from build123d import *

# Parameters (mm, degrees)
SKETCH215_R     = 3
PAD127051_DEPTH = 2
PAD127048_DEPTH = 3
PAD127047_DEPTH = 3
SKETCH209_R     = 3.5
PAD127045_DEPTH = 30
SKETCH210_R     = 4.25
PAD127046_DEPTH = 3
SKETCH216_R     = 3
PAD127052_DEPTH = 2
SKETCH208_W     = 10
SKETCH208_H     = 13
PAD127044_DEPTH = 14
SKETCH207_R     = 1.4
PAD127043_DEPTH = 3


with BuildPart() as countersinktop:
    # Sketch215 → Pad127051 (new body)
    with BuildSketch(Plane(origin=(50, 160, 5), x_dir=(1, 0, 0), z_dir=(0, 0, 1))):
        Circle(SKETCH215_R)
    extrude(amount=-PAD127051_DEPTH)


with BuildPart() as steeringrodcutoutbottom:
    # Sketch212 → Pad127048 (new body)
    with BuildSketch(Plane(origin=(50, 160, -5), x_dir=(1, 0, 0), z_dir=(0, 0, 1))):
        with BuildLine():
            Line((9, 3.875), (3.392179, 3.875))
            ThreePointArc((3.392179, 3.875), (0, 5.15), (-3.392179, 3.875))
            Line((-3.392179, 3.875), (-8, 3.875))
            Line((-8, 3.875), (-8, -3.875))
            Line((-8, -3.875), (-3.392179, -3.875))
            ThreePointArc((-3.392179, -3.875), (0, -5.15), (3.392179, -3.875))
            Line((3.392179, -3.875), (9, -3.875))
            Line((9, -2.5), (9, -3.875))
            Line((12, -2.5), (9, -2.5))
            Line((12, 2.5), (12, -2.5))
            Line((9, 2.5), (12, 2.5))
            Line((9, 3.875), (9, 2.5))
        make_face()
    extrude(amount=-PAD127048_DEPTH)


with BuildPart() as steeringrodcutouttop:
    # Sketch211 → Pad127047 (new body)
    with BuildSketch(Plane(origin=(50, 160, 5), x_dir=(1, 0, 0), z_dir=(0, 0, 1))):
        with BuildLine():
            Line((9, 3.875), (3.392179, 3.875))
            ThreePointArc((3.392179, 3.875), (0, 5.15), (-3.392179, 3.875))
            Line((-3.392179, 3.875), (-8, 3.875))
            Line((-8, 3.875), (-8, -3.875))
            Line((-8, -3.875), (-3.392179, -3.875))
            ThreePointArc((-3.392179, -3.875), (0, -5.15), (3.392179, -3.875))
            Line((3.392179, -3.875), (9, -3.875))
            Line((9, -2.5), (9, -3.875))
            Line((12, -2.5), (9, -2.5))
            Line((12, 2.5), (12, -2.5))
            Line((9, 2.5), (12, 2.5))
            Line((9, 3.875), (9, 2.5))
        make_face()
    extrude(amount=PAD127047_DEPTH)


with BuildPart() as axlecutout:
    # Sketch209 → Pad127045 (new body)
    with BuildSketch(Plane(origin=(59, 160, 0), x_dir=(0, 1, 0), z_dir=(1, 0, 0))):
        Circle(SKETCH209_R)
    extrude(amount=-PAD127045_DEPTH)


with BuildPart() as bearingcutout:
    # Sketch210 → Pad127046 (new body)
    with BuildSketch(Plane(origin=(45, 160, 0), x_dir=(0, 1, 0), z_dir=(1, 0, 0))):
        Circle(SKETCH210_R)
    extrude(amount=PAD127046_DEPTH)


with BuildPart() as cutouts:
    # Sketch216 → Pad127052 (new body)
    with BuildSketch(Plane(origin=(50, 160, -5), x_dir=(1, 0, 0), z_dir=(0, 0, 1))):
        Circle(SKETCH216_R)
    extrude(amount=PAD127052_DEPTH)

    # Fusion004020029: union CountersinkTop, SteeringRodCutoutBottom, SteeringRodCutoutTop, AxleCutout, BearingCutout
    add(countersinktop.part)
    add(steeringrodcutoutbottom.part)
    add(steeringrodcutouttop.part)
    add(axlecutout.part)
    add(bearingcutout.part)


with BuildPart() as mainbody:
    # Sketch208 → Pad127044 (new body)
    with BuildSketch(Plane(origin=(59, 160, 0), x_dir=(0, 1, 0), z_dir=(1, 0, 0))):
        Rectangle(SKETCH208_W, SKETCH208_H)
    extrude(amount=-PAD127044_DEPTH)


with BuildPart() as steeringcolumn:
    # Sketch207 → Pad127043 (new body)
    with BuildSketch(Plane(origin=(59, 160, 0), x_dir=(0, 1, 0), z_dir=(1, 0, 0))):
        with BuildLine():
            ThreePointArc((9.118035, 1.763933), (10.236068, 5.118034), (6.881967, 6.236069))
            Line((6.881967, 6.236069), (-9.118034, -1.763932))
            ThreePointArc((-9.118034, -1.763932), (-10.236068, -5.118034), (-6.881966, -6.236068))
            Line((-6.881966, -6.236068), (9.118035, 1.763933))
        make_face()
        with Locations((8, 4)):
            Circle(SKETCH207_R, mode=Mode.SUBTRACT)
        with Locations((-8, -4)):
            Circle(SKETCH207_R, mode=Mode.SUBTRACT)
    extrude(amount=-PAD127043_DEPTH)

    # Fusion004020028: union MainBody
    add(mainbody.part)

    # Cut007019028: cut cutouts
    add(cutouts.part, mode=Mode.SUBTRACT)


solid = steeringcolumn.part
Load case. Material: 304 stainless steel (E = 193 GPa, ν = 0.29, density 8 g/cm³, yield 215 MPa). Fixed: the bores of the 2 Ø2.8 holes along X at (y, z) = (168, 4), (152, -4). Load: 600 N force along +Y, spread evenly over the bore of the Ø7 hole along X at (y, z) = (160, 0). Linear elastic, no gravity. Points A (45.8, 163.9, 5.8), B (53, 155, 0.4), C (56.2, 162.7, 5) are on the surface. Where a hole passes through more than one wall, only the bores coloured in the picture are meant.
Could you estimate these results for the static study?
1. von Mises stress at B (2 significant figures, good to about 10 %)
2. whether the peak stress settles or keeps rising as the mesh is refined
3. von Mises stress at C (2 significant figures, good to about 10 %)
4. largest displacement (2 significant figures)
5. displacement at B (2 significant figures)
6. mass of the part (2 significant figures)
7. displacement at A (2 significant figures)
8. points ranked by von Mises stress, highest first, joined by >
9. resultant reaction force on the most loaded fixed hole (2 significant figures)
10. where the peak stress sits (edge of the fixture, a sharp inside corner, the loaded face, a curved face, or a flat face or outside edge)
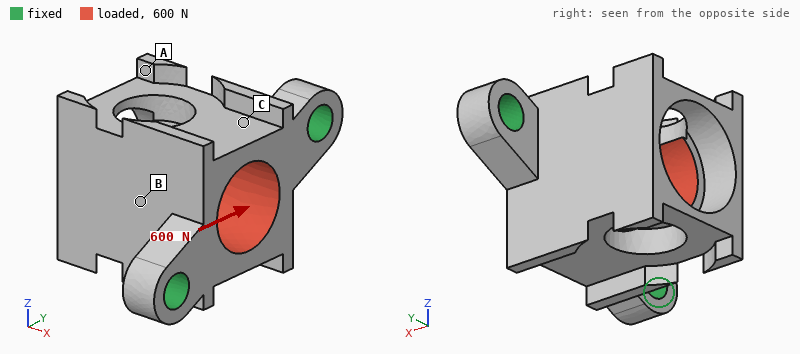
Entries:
19 MPa
keeps rising
40 MPa
12 µm
5.1 µm
7.2 g
10 µm
C > B > A
330 N
edge of the fixture
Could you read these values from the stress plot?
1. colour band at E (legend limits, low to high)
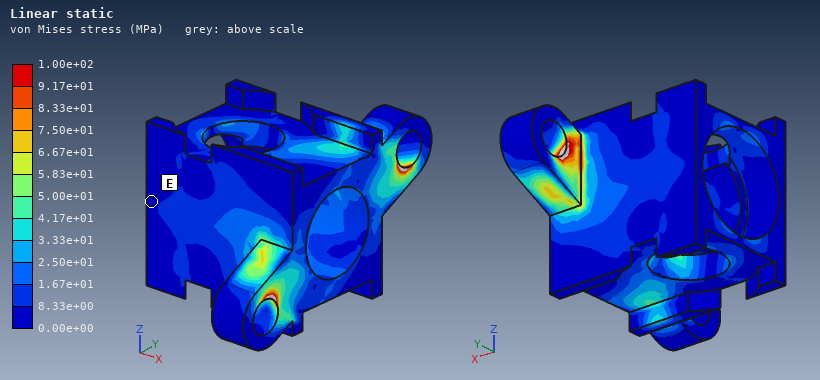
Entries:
0.00e+00 to 8.33e+00 MPa
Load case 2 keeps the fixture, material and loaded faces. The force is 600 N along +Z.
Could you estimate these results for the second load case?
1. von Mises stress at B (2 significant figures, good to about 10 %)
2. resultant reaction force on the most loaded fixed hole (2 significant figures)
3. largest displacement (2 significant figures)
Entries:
13 MPa
310 N
20 µm
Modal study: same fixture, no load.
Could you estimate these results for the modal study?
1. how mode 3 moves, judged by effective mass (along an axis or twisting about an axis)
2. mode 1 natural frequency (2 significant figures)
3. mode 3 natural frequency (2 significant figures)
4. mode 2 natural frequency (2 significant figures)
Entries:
along X
10 kHz
26 kHz
25 kHz
